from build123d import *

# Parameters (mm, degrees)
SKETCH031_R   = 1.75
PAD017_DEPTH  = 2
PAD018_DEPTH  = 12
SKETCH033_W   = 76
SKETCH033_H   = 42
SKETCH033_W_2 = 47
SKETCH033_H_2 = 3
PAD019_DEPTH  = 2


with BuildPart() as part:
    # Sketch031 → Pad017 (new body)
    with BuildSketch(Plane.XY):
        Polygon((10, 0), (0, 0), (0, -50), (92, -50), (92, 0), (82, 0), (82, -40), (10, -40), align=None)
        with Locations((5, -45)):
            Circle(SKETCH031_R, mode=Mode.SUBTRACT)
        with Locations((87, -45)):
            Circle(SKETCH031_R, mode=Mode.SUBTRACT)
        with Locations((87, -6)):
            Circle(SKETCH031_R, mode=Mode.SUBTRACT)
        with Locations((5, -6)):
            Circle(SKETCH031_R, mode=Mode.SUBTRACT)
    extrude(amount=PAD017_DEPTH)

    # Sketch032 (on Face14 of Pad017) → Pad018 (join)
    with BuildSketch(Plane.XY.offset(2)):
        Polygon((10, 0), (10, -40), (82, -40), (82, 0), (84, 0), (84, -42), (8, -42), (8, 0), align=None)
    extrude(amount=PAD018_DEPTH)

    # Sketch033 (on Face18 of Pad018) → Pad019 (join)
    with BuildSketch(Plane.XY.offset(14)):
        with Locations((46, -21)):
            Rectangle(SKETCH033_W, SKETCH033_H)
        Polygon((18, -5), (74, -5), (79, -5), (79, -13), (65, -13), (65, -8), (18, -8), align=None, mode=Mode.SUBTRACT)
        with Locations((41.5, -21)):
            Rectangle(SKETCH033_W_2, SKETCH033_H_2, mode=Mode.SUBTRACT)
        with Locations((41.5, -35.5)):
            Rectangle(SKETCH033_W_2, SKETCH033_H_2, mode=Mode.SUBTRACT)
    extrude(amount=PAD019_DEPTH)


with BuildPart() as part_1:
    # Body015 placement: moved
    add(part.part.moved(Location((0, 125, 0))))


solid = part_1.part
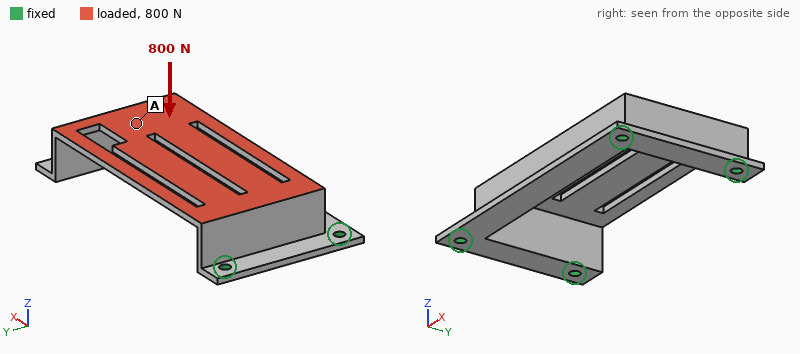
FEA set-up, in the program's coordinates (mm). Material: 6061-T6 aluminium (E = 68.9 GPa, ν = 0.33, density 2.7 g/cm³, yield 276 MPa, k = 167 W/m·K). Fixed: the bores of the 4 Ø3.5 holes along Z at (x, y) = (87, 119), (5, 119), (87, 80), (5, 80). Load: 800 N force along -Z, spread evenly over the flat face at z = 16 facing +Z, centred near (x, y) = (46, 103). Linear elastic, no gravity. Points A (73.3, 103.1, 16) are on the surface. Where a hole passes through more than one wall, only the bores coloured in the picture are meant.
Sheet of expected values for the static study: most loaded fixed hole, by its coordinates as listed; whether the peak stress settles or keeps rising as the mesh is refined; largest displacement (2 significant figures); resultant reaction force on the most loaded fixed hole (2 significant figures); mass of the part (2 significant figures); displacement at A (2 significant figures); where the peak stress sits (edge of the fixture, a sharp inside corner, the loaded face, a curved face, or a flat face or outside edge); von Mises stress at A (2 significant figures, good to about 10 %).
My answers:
(5, 119)
keeps rising
0.55 mm
350 N
34 g
0.097 mm
a sharp inside corner
71 MPa
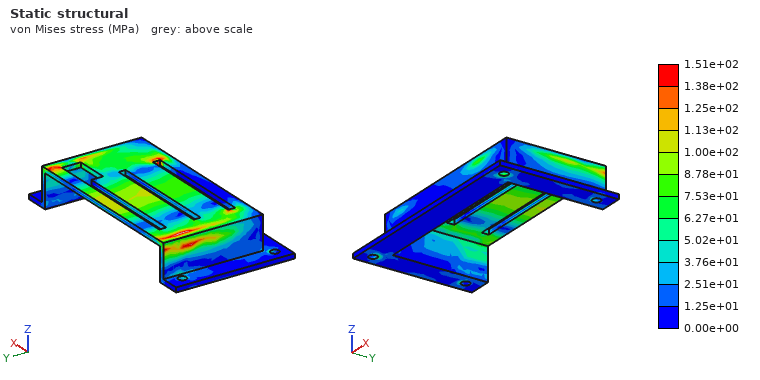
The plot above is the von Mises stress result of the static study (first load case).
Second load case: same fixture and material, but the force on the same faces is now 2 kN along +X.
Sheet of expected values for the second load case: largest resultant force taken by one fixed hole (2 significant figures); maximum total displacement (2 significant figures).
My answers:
1.0 kN
0.15 mm
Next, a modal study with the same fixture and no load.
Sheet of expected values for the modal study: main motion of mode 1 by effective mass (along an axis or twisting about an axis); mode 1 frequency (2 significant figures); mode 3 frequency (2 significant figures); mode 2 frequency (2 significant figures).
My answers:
along Z
1900 Hz
3100 Hz
2200 Hz
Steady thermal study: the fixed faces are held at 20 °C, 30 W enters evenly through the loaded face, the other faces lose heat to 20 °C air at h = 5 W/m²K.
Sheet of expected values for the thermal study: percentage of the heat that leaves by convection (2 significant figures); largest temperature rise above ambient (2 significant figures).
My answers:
3.3 %
42 K
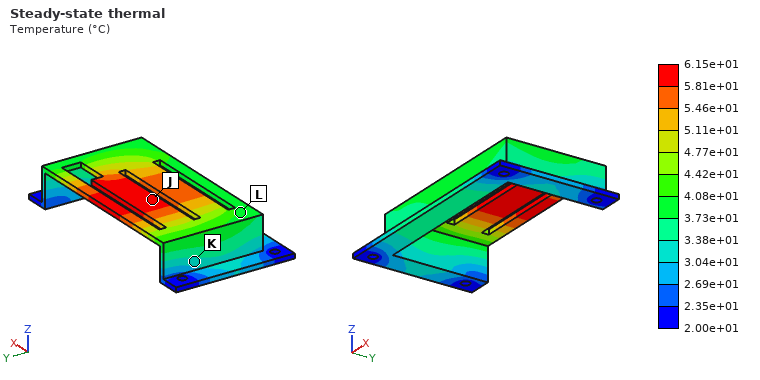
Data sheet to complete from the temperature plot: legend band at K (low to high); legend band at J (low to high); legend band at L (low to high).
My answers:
3.04e+01 to 3.38e+01 °C
5.81e+01 to 6.15e+01 °C
3.73e+01 to 4.08e+01 °C
